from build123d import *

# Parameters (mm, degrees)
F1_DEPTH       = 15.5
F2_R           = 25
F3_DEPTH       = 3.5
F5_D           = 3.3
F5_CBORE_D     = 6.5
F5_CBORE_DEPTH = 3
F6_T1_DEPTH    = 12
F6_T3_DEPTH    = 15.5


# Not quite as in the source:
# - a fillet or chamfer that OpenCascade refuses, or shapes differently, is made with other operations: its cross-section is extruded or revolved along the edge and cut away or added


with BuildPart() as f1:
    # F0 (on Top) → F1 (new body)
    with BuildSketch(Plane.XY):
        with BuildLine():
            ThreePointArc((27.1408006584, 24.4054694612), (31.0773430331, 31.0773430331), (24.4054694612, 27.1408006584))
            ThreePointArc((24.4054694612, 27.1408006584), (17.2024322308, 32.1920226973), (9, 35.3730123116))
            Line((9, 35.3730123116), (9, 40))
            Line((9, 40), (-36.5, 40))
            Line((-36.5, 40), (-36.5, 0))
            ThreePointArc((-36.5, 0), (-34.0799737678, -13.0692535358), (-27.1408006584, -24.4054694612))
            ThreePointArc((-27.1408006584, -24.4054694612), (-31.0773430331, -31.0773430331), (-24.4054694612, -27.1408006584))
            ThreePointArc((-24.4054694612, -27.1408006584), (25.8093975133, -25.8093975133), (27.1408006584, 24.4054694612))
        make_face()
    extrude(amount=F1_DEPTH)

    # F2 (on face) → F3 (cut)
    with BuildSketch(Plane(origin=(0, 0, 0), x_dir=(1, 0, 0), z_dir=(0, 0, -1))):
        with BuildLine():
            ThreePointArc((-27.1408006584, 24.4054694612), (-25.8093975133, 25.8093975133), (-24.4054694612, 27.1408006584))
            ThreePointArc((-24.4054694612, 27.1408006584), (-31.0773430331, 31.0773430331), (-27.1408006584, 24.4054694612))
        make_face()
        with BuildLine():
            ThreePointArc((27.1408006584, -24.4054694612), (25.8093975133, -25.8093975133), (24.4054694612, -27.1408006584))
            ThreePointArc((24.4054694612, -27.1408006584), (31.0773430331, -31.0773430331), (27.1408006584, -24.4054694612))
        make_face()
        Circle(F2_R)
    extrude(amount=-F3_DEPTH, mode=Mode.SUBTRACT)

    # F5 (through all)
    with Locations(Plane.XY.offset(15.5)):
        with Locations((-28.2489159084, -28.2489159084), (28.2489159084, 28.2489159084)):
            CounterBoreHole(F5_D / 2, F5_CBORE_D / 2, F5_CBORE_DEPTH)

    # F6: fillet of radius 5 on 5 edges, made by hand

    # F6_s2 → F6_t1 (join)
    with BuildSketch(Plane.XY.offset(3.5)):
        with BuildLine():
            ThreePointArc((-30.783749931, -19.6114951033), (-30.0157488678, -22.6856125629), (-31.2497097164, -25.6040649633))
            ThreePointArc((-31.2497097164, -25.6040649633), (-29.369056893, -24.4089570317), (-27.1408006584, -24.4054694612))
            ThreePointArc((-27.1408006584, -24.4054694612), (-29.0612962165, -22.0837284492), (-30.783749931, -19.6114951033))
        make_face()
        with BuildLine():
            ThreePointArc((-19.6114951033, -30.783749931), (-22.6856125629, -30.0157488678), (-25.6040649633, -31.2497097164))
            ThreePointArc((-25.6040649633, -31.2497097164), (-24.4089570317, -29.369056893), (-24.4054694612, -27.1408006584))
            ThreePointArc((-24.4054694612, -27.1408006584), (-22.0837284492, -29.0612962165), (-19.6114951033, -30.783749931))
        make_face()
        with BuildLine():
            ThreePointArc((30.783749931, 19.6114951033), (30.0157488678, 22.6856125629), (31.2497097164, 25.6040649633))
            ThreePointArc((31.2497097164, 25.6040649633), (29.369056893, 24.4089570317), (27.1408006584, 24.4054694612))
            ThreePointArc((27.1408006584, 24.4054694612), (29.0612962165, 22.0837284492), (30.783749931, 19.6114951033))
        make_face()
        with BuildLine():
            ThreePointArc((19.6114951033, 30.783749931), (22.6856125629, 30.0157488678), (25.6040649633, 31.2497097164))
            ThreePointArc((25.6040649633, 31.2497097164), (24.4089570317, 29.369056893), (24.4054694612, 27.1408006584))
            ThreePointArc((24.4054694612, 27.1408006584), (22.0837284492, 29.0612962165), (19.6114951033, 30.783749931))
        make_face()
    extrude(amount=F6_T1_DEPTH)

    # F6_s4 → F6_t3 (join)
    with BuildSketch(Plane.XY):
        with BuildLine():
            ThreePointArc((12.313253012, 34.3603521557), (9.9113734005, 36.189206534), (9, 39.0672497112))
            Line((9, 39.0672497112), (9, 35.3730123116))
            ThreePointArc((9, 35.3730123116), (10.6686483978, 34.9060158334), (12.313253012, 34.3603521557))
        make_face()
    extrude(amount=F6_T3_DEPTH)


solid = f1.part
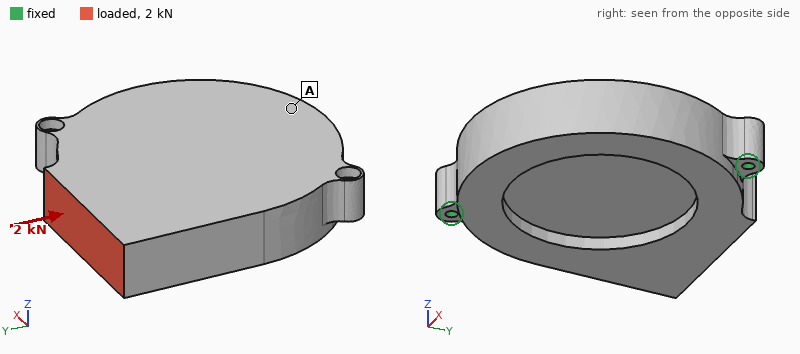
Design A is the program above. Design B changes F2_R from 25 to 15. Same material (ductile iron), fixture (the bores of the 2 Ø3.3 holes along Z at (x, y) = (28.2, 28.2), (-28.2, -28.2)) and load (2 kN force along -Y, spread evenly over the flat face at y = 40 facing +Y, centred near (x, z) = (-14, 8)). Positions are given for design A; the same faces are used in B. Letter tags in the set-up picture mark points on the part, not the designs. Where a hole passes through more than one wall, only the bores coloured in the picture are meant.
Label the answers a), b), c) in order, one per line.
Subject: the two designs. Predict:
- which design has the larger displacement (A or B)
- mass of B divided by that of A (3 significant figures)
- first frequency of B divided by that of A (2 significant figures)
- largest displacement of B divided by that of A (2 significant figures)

a) A
b) 1.07
c) 0.99
d) 0.91
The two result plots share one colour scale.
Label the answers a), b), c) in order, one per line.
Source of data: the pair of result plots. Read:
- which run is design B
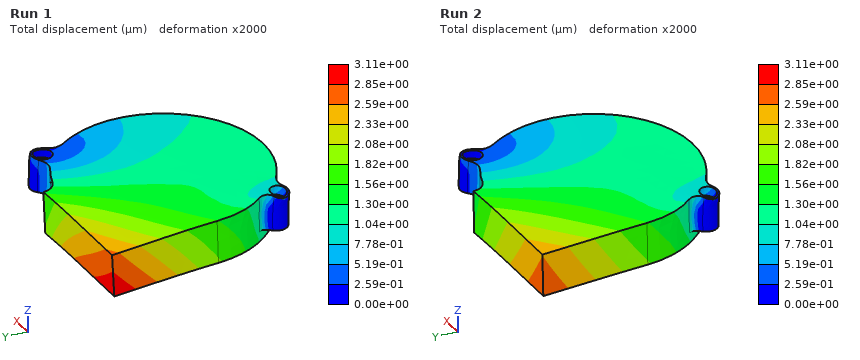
a) Run 2
